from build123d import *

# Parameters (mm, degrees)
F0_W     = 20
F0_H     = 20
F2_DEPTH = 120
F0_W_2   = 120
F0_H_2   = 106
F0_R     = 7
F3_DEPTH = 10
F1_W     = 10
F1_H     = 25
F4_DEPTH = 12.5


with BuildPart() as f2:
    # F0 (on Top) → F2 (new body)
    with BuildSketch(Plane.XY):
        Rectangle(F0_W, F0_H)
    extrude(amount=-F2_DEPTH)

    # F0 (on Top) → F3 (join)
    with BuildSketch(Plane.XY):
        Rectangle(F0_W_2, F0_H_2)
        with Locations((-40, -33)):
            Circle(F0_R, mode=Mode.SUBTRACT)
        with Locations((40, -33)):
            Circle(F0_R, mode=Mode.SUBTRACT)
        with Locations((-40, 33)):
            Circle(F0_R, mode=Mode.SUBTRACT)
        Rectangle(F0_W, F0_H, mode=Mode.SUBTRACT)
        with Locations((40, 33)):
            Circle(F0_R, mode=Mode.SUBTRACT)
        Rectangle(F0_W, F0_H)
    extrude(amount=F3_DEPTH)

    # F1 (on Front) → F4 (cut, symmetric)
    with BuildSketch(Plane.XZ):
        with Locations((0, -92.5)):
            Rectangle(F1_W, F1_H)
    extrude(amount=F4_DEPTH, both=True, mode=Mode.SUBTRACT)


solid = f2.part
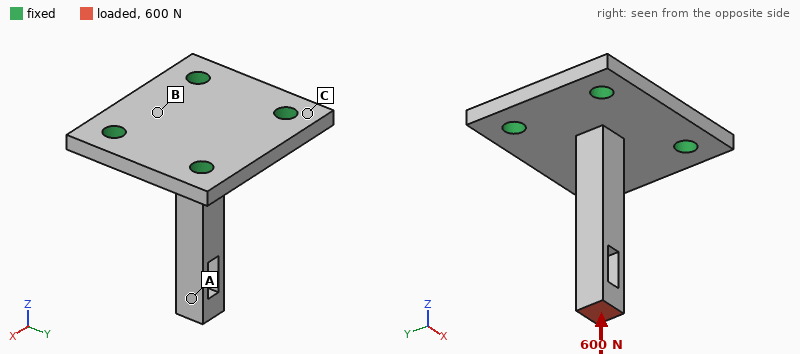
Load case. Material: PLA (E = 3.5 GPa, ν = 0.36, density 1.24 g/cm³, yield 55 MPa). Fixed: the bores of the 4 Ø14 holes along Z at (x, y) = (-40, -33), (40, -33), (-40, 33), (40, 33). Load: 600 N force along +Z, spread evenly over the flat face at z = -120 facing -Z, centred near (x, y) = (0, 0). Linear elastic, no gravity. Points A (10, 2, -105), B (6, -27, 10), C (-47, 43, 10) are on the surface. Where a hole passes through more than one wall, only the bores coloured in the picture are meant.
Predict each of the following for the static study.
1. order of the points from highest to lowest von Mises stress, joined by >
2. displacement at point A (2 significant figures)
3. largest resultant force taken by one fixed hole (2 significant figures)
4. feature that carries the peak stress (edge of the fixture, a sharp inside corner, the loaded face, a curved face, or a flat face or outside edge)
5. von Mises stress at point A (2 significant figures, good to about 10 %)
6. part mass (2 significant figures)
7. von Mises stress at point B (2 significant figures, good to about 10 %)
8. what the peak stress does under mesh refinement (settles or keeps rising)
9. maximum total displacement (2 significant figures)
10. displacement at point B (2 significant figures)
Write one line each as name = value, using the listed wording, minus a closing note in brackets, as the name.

order of the points from highest to lowest von Mises stress, joined by > = A > B > C
displacement at point A = 0.14 mm
largest resultant force taken by one fixed hole = 150 N
feature that carries the peak stress = edge of the fixture
von Mises stress at point A = 2.8 MPa
part mass = 200 g
von Mises stress at point B = 1.7 MPa
what the peak stress does under mesh refinement = keeps rising
maximum total displacement = 0.15 mm
displacement at point B = 0.045 mm
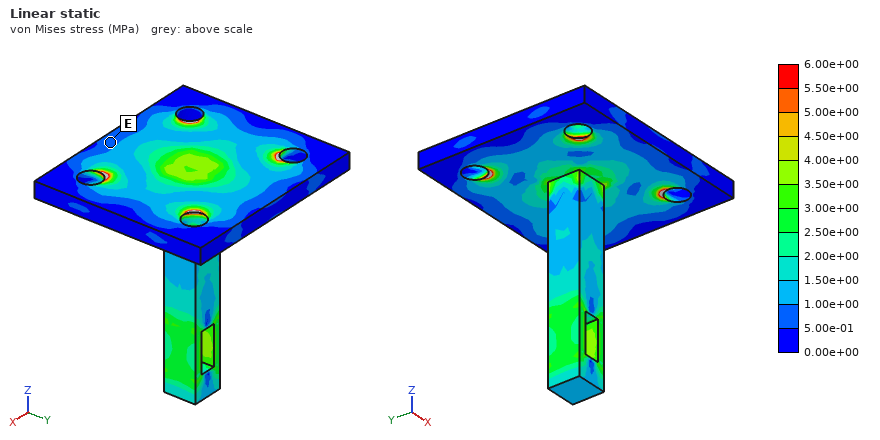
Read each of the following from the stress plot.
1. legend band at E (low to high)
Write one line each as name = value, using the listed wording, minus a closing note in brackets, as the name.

legend band at E = 5.00e-01 to 1.00e+00 MPa
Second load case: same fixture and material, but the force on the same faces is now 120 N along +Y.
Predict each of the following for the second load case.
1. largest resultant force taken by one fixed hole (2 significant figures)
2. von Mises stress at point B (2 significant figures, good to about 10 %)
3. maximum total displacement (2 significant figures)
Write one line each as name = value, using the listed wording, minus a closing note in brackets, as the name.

largest resultant force taken by one fixed hole = 140 N
von Mises stress at point B = 2.0 MPa
maximum total displacement = 2.2 mm
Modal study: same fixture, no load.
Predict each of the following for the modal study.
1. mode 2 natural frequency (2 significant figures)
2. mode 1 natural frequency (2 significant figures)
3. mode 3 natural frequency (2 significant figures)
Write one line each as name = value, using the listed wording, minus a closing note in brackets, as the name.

mode 2 natural frequency = 330 Hz
mode 1 natural frequency = 330 Hz
mode 3 natural frequency = 1500 Hz
